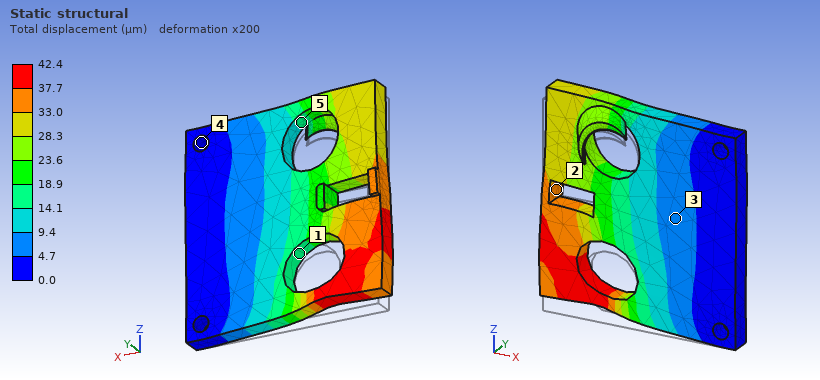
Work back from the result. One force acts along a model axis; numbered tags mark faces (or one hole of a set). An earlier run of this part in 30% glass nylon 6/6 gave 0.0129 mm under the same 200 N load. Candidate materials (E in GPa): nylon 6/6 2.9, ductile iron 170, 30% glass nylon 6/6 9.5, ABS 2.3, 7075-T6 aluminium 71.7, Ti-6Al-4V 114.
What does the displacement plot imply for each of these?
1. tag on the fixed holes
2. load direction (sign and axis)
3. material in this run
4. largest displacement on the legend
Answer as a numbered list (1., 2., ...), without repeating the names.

1. 4
2. +Z
3. nylon 6/6
4. 42.4 µm
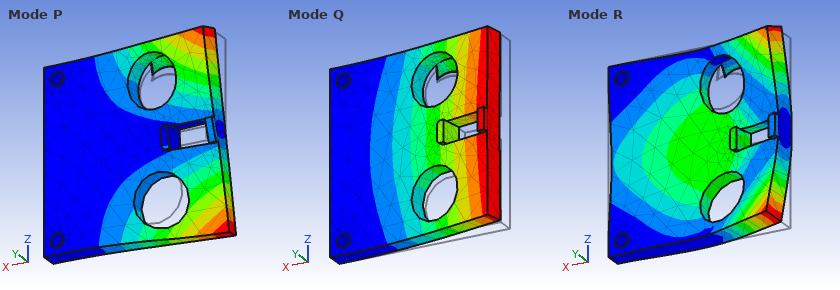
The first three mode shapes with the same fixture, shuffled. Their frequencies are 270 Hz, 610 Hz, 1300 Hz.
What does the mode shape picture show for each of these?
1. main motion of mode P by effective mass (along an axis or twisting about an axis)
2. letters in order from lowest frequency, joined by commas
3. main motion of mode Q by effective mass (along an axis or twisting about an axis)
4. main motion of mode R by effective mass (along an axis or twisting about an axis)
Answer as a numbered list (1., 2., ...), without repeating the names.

1. twisting about X
2. Q, P, R
3. along Y
4. along Y
